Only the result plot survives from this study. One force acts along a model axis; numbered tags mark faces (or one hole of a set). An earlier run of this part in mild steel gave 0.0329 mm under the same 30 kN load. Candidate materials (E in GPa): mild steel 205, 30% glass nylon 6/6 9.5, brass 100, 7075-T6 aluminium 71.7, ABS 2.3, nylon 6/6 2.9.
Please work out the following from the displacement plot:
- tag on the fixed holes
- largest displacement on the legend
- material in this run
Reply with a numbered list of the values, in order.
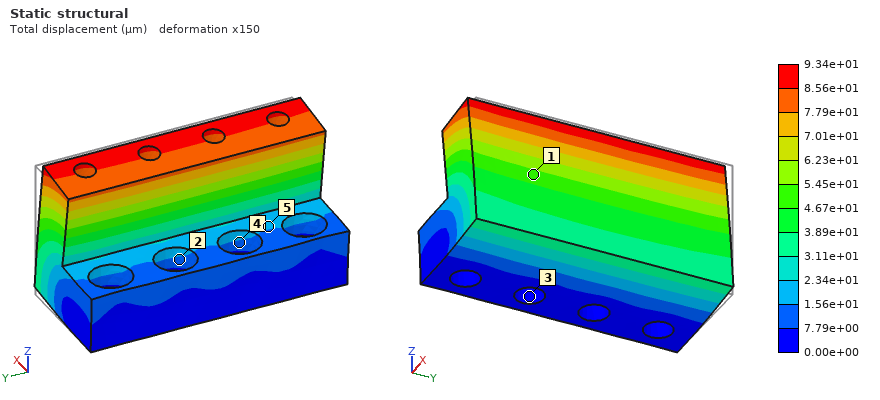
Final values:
1. 3
2. 9.34e+01 µm
3. 7075-T6 aluminium
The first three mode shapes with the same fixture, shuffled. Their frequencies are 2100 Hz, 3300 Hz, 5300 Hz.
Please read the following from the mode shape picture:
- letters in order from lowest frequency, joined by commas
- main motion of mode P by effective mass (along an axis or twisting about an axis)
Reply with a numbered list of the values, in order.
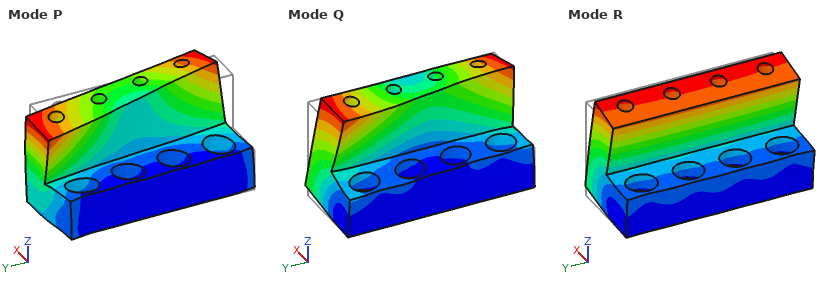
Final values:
1. R, Q, P
2. along Y
